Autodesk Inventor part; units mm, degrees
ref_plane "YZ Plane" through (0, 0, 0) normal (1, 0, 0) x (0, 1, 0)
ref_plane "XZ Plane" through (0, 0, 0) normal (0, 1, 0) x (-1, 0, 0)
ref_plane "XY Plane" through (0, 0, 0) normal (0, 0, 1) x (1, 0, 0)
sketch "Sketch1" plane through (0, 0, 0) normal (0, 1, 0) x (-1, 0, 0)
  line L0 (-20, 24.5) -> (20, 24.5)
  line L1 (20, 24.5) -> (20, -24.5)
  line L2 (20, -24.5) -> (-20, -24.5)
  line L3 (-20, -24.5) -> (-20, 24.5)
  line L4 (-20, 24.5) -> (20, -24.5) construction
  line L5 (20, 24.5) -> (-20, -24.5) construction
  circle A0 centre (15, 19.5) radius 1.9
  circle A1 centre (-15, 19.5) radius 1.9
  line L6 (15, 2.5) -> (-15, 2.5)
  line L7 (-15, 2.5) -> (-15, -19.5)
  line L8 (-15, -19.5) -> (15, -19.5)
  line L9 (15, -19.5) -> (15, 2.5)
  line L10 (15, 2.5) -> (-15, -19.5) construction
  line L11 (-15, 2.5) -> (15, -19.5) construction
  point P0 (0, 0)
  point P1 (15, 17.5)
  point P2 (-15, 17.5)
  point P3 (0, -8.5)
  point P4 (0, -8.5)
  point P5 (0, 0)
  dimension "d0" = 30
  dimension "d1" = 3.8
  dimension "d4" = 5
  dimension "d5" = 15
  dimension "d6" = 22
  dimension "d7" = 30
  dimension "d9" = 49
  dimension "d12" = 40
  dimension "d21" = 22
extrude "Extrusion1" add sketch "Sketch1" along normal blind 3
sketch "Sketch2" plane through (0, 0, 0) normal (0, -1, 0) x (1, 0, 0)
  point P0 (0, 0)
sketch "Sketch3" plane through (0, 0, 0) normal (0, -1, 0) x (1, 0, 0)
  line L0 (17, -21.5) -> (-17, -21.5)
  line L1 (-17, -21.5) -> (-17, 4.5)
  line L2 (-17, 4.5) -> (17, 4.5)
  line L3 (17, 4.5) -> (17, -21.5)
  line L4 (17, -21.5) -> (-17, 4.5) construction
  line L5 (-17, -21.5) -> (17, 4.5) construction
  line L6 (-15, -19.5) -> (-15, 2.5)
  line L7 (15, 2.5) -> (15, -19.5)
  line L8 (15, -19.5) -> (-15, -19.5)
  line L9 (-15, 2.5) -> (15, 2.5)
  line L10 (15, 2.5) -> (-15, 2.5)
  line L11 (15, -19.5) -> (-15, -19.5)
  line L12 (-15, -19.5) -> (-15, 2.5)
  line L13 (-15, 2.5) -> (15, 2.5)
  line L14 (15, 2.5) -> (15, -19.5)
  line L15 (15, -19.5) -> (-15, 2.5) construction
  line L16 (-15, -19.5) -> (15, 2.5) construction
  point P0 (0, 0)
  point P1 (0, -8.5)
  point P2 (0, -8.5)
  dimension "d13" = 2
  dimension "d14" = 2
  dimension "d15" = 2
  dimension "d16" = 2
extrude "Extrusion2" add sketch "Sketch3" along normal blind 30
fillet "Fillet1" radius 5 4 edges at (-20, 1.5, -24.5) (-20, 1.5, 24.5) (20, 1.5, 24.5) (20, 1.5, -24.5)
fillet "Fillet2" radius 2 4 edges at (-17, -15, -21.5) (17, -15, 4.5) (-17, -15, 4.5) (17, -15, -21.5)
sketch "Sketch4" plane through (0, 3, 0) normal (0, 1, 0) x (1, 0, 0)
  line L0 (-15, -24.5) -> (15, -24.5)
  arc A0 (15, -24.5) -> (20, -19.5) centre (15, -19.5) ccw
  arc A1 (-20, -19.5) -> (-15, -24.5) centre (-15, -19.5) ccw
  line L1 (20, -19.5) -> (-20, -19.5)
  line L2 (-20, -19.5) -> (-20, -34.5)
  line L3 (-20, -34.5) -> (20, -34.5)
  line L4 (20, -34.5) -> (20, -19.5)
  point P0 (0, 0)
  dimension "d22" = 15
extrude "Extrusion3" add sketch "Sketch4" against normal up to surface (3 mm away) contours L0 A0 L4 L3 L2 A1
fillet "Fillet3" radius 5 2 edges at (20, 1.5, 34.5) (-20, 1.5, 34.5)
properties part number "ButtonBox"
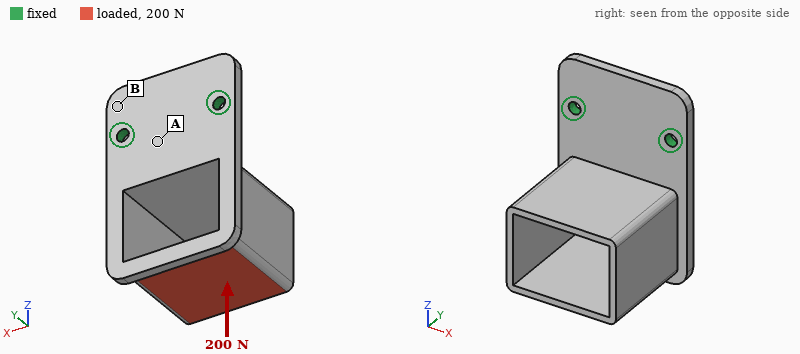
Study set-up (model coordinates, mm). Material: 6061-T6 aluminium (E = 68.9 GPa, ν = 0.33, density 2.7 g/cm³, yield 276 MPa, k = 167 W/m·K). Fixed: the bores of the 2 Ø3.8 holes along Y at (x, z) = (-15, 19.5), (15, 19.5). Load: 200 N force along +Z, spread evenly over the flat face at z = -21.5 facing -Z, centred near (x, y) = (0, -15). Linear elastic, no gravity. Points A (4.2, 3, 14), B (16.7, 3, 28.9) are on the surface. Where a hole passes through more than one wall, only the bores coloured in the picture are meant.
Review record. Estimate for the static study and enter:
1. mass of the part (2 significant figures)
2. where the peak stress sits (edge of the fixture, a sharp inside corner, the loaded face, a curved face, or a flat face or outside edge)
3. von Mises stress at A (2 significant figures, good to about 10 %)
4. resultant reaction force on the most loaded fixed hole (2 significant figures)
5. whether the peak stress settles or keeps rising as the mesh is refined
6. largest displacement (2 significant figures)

31 g
edge of the fixture
38 MPa
100 N
keeps rising
0.54 mm
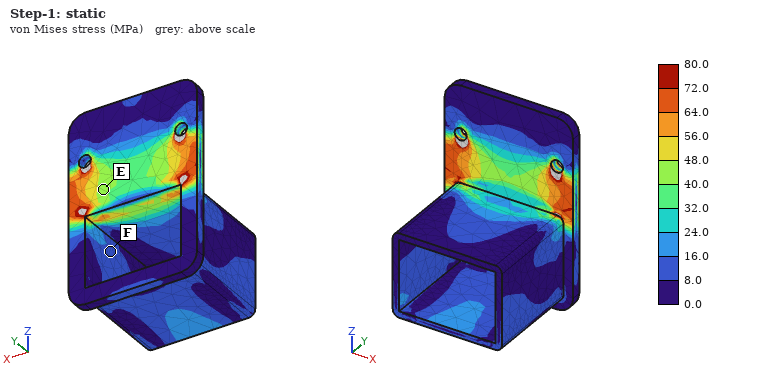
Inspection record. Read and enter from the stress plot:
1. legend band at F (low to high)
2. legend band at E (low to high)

8.0 to 16.0 MPa
40.0 to 48.0 MPa
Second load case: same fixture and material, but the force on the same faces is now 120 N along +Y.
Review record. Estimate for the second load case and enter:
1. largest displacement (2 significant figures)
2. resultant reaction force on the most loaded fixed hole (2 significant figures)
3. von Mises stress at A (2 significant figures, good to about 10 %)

0.60 mm
64 N
47 MPa
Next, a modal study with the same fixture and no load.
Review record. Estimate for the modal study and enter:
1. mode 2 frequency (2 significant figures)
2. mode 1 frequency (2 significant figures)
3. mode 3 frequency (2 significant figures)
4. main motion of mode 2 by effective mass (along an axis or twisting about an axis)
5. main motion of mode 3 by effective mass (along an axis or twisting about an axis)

1900 Hz
660 Hz
2900 Hz
along X
along X
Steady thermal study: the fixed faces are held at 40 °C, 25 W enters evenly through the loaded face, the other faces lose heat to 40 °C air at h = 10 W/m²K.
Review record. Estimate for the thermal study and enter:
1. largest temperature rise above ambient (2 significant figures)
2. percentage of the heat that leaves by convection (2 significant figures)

64 K
13 %
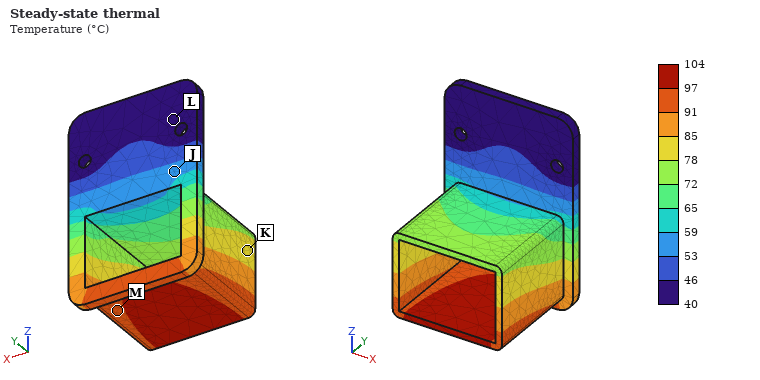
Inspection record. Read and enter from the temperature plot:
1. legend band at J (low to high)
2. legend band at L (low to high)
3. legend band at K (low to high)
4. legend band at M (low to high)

53 to 59 °C
40 to 46 °C
78 to 85 °C
91 to 97 °C
